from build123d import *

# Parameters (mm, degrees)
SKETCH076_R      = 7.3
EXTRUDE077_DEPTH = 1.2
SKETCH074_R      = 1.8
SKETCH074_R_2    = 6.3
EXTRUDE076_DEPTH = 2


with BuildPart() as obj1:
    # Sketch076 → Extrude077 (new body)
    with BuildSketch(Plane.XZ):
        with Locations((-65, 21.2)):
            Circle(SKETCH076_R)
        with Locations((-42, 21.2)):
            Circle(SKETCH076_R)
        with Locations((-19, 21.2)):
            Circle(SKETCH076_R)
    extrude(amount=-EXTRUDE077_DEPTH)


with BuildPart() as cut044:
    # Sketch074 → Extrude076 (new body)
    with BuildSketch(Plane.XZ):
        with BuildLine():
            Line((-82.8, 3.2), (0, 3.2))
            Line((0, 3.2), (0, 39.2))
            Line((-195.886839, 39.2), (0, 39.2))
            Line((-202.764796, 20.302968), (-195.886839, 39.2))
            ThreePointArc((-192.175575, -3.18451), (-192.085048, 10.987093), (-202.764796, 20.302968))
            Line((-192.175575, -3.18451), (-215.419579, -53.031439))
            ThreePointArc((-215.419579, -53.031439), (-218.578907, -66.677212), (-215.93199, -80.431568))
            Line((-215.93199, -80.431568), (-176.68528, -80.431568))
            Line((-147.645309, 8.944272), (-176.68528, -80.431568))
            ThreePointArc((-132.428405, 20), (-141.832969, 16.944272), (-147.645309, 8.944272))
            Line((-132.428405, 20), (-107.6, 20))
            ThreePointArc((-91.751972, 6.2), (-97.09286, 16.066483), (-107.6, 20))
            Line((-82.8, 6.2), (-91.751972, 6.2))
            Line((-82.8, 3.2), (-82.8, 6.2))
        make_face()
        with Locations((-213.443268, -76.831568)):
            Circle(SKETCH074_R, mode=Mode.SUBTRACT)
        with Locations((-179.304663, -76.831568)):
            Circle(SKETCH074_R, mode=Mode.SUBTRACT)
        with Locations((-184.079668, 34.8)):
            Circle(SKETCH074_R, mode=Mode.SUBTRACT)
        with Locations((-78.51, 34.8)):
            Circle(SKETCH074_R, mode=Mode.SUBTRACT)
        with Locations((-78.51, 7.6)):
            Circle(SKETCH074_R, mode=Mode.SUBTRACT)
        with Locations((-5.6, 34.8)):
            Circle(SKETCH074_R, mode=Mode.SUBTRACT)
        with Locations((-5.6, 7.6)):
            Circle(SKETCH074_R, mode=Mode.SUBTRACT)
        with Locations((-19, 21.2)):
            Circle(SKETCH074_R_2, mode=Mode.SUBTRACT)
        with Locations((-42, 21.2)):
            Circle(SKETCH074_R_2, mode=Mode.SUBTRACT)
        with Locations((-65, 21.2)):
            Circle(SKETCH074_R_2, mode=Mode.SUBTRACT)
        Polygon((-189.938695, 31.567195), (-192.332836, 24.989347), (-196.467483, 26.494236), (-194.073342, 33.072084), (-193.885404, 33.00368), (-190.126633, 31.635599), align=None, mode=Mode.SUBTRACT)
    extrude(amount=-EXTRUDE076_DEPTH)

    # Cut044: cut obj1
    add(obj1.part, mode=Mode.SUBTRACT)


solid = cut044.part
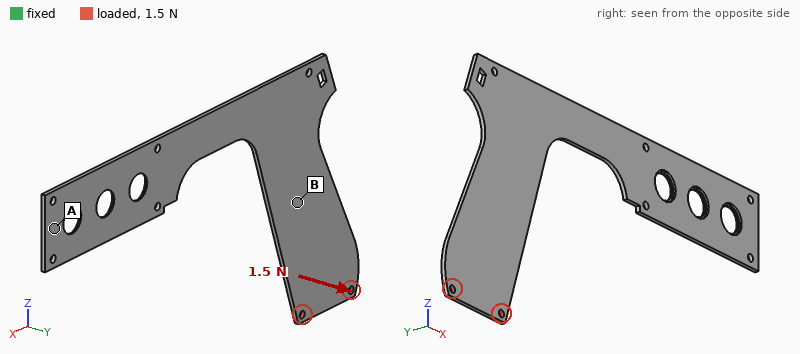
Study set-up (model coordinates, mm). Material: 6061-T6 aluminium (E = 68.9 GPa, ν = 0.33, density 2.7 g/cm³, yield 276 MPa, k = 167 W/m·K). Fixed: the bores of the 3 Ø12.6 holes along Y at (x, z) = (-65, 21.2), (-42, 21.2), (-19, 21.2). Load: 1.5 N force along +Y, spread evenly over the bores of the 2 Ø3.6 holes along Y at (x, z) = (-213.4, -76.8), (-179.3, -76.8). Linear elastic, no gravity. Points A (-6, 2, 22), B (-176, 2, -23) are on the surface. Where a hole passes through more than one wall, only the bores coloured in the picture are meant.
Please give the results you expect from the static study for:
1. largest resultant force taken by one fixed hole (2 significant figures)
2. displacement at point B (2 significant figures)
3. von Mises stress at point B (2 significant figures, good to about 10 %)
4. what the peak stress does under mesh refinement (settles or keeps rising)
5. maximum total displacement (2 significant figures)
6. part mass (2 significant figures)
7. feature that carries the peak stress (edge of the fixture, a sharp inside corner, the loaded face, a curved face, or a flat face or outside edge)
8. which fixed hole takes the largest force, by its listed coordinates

16 N
1.2 mm
3.2 MPa
keeps rising
2.5 mm
51 g
edge of the fixture
(-65, 21.2)
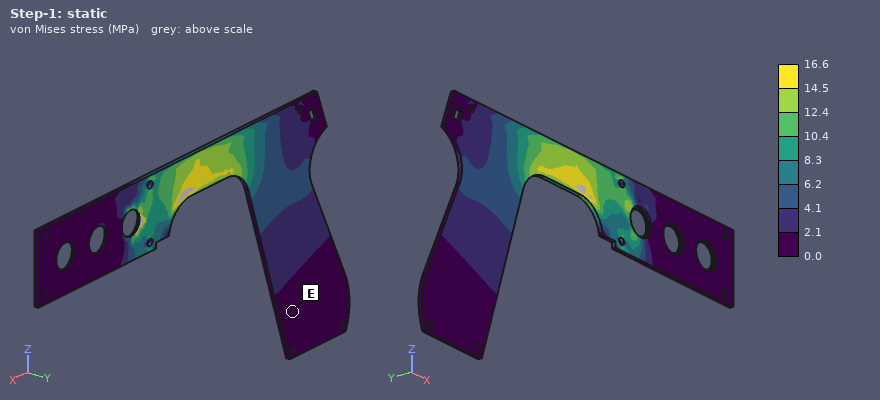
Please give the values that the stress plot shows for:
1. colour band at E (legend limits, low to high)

0.0 to 2.1 MPa
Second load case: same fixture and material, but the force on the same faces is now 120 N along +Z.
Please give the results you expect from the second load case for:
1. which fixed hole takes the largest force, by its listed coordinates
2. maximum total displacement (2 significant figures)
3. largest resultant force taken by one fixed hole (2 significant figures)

(-65, 21.2)
1.2 mm
390 N
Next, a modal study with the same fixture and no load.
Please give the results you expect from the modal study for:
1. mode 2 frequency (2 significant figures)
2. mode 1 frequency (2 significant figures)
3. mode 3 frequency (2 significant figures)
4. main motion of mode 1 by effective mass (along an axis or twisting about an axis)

120 Hz
37 Hz
360 Hz
along Y
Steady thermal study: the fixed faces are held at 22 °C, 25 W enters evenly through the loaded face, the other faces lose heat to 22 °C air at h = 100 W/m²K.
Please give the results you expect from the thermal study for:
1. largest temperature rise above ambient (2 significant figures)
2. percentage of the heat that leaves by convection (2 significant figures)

81 K
99 %
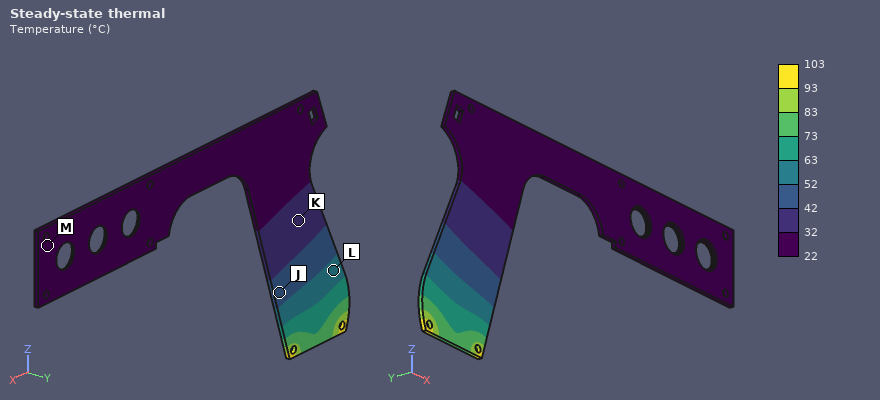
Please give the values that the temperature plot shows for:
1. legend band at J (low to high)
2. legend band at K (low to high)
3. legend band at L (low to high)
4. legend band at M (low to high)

42 to 52 °C
32 to 42 °C
52 to 63 °C
22 to 32 °C
